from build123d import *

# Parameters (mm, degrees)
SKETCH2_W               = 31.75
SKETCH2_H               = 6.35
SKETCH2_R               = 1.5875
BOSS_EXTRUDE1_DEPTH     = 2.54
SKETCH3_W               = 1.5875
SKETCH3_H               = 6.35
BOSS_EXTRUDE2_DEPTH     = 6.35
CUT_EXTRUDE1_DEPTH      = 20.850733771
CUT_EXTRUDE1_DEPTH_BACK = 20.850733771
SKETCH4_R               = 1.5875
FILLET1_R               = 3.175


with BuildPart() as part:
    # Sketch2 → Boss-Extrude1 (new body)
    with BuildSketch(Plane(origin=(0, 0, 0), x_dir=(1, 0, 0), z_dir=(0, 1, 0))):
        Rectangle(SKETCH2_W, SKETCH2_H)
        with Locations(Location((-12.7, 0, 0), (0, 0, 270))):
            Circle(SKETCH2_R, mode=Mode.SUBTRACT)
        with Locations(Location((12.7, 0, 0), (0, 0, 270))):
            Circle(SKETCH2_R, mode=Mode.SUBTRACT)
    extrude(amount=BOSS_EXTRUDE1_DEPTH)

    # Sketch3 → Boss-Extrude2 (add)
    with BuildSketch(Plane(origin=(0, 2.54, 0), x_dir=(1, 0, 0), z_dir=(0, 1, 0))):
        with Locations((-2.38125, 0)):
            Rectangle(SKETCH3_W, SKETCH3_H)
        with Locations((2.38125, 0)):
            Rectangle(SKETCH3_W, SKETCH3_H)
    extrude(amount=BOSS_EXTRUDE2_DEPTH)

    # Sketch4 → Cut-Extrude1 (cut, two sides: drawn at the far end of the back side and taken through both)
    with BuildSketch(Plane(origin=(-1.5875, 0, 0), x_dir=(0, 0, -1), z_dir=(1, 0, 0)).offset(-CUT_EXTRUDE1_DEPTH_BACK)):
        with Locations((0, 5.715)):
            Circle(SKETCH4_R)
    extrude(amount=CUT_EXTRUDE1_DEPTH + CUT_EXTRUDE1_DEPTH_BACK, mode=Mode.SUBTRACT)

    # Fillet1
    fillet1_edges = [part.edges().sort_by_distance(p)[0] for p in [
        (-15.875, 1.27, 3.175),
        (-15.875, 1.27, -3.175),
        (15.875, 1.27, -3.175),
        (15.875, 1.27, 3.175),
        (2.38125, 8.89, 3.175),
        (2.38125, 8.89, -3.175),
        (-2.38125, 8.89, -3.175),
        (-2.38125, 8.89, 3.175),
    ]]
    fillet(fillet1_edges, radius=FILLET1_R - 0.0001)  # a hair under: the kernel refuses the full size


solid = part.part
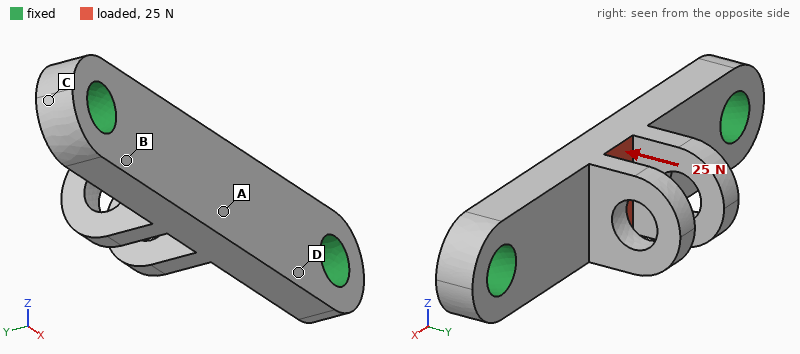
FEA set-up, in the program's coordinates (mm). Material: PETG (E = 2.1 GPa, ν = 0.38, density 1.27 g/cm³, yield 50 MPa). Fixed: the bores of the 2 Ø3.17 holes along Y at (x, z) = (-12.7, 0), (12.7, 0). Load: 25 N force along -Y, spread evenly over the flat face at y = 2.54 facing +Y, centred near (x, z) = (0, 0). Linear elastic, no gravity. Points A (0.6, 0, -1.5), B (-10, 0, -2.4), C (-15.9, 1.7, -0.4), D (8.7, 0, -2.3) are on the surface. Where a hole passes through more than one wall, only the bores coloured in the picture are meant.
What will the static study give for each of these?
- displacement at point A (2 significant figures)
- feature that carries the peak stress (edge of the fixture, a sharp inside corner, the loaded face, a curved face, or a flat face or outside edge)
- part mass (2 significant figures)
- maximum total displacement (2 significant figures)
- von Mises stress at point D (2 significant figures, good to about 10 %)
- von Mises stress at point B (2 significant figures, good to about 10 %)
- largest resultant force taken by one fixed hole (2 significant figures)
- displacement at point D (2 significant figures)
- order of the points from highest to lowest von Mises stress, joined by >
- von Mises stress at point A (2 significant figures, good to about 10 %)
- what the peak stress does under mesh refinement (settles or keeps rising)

0.092 mm
edge of the fixture
0.68 g
0.11 mm
4.8 MPa
6.0 MPa
13 N
0.020 mm
A > B > D > C
8.5 MPa
keeps rising
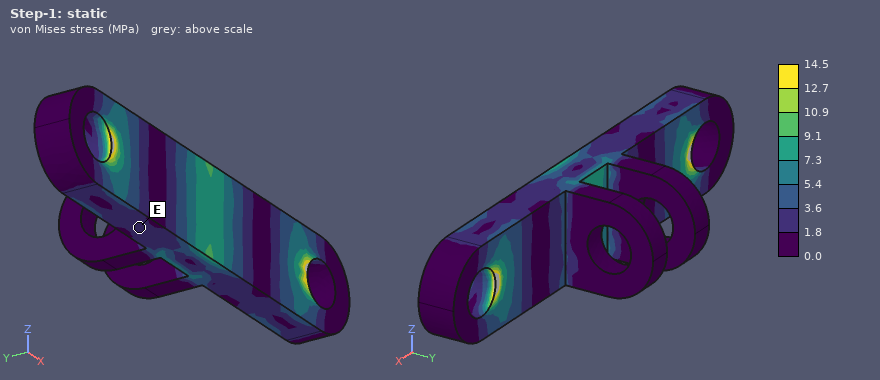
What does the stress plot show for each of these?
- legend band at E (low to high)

1.8 to 3.6 MPa
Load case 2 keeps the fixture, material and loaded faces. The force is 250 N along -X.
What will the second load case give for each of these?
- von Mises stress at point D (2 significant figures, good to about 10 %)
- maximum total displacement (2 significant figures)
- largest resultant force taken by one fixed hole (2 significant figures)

8.6 MPa
0.11 mm
130 N
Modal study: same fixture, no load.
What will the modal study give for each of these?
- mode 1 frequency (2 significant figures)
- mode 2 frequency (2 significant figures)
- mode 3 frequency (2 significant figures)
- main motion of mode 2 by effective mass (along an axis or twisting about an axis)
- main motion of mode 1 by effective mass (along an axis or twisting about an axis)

4700 Hz
5300 Hz
7200 Hz
along Z
along Y
